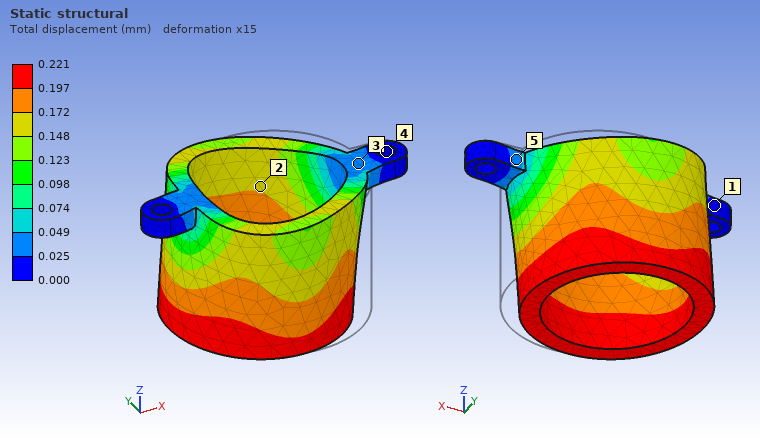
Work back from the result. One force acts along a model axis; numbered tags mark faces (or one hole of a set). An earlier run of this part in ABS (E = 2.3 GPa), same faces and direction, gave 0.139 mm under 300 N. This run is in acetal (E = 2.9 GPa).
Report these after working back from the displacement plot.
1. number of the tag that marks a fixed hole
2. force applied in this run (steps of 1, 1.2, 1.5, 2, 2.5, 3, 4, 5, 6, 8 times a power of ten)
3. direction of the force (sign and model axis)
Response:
4
600 N
-X
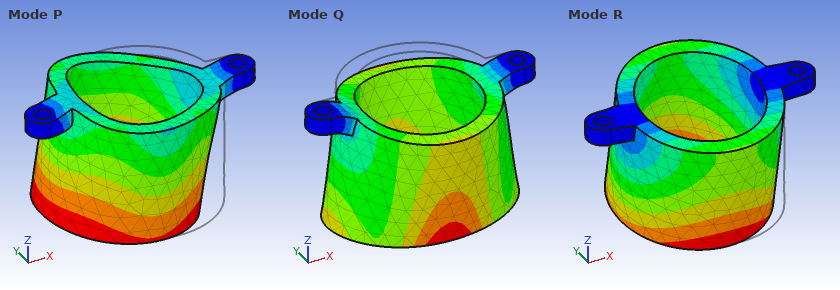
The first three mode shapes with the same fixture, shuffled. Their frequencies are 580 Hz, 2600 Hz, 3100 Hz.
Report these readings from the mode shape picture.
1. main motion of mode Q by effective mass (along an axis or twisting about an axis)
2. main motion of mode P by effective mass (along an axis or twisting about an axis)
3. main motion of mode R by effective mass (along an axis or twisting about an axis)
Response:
along Z
along X
along Y
